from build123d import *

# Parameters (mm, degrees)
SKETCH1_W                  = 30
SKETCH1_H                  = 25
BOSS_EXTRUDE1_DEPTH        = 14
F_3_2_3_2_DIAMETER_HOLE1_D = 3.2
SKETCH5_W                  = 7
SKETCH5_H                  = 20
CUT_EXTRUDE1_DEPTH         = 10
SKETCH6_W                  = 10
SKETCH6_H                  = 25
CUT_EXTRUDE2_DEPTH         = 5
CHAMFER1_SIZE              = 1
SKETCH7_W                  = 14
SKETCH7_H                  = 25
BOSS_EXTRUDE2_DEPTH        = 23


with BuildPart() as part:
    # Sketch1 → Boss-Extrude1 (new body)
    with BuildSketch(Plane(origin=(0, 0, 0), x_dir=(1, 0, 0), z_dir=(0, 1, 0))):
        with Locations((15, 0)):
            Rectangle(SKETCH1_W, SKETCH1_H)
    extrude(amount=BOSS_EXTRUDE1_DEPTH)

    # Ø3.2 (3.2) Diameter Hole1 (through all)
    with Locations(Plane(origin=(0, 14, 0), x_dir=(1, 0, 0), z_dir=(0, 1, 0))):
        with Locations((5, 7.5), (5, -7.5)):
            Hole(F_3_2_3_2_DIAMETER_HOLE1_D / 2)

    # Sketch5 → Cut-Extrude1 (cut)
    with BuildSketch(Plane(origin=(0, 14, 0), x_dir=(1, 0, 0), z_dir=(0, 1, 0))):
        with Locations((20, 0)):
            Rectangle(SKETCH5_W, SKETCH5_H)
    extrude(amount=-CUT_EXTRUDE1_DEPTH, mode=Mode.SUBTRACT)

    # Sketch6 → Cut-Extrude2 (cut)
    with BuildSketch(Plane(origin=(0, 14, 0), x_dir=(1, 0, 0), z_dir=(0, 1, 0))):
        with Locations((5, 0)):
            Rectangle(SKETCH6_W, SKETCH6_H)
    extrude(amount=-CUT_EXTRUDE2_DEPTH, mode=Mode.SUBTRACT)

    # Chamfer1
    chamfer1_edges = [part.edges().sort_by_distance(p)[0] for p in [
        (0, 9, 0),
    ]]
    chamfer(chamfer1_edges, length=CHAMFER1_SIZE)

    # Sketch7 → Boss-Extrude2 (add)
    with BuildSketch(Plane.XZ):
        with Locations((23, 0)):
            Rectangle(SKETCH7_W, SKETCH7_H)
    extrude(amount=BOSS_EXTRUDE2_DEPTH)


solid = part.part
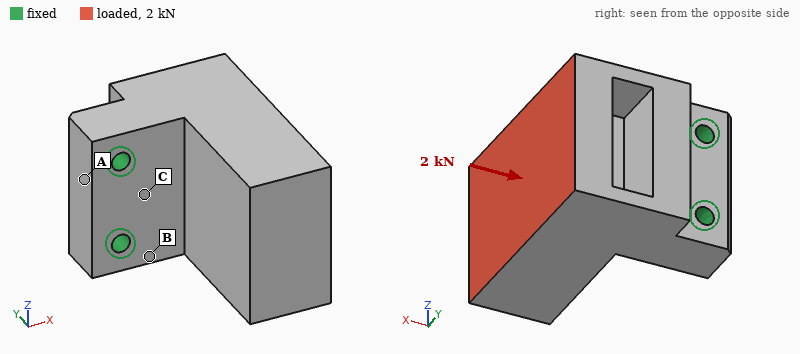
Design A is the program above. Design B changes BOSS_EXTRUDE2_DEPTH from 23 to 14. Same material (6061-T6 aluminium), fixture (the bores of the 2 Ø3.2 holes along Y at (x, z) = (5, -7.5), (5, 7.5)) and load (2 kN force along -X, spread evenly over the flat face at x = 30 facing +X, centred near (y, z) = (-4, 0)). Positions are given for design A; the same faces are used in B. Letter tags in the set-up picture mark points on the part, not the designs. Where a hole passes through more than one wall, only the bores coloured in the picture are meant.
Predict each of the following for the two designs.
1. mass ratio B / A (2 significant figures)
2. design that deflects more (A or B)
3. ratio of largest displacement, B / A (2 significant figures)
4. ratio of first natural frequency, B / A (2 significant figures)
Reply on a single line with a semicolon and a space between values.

0.80; A; 0.38; 1.4
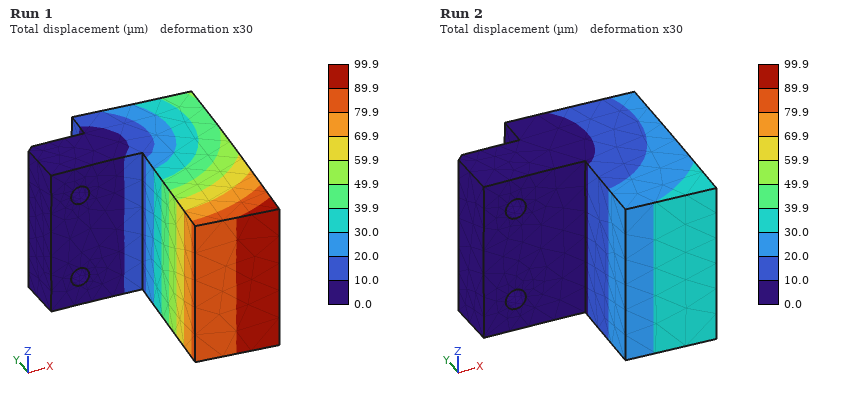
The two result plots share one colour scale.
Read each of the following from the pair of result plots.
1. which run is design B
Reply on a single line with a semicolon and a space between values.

Run 2
